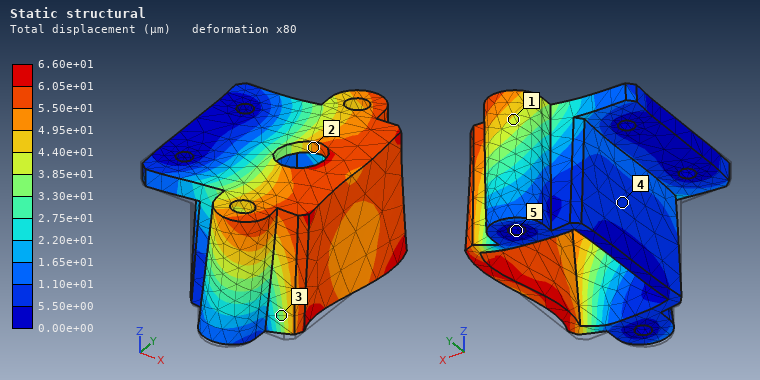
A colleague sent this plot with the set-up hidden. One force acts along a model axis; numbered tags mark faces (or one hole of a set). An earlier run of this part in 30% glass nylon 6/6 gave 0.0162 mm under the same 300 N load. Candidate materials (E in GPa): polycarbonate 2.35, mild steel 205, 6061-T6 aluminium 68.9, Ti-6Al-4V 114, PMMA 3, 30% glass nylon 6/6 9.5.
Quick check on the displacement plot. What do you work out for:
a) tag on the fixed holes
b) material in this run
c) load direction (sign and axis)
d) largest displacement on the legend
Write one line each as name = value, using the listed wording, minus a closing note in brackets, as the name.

tag on the fixed holes = 5
material in this run = polycarbonate
load direction = +Y
largest displacement on the legend = 6.60e+01 µm
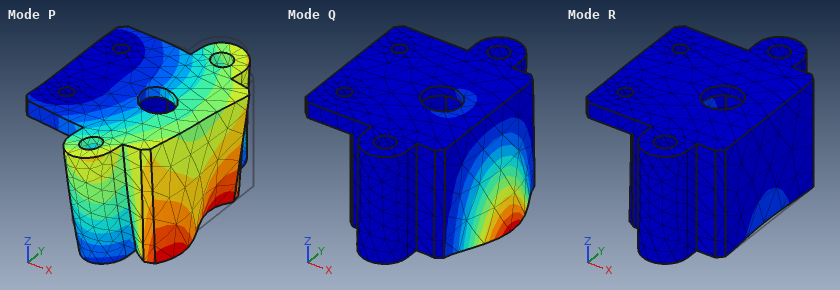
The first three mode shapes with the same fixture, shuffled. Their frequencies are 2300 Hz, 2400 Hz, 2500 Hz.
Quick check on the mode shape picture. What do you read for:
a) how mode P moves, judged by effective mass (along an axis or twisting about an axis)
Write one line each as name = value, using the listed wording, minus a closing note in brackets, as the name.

how mode P moves, judged by effective mass = along Y
